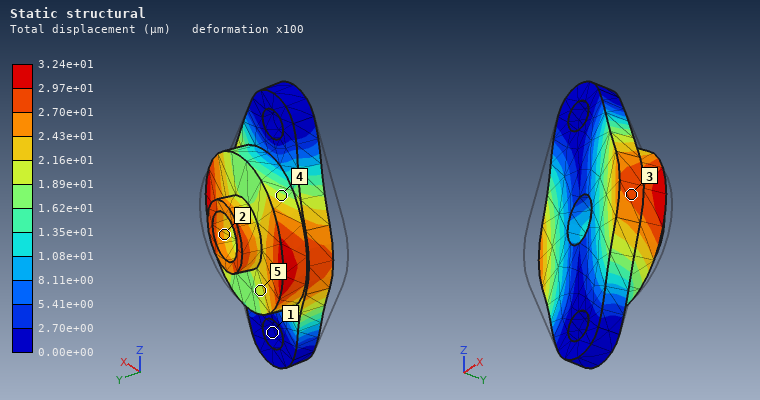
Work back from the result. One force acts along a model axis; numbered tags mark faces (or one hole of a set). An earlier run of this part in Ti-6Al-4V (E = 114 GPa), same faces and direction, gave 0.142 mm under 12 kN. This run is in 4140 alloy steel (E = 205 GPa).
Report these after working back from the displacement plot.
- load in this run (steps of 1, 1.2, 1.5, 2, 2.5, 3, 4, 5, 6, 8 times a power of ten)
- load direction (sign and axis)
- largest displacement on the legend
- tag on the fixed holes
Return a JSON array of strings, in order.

["5 kN", "+X", "3.24e+01 µm", "1"]
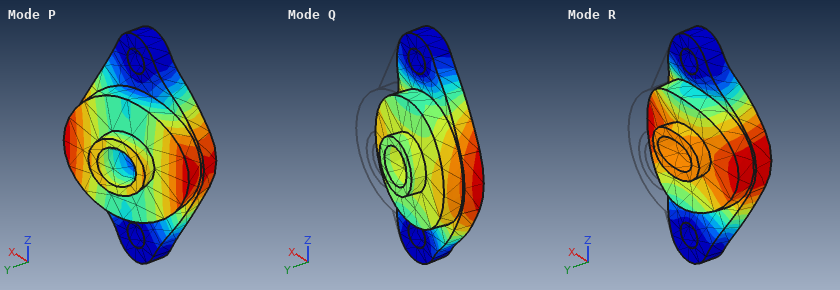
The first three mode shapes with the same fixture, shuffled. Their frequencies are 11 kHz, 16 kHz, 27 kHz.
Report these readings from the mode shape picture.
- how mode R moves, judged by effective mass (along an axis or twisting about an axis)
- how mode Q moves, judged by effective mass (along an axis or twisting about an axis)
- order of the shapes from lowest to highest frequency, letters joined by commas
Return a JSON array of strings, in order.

["along Y", "along X", "P, R, Q"]
